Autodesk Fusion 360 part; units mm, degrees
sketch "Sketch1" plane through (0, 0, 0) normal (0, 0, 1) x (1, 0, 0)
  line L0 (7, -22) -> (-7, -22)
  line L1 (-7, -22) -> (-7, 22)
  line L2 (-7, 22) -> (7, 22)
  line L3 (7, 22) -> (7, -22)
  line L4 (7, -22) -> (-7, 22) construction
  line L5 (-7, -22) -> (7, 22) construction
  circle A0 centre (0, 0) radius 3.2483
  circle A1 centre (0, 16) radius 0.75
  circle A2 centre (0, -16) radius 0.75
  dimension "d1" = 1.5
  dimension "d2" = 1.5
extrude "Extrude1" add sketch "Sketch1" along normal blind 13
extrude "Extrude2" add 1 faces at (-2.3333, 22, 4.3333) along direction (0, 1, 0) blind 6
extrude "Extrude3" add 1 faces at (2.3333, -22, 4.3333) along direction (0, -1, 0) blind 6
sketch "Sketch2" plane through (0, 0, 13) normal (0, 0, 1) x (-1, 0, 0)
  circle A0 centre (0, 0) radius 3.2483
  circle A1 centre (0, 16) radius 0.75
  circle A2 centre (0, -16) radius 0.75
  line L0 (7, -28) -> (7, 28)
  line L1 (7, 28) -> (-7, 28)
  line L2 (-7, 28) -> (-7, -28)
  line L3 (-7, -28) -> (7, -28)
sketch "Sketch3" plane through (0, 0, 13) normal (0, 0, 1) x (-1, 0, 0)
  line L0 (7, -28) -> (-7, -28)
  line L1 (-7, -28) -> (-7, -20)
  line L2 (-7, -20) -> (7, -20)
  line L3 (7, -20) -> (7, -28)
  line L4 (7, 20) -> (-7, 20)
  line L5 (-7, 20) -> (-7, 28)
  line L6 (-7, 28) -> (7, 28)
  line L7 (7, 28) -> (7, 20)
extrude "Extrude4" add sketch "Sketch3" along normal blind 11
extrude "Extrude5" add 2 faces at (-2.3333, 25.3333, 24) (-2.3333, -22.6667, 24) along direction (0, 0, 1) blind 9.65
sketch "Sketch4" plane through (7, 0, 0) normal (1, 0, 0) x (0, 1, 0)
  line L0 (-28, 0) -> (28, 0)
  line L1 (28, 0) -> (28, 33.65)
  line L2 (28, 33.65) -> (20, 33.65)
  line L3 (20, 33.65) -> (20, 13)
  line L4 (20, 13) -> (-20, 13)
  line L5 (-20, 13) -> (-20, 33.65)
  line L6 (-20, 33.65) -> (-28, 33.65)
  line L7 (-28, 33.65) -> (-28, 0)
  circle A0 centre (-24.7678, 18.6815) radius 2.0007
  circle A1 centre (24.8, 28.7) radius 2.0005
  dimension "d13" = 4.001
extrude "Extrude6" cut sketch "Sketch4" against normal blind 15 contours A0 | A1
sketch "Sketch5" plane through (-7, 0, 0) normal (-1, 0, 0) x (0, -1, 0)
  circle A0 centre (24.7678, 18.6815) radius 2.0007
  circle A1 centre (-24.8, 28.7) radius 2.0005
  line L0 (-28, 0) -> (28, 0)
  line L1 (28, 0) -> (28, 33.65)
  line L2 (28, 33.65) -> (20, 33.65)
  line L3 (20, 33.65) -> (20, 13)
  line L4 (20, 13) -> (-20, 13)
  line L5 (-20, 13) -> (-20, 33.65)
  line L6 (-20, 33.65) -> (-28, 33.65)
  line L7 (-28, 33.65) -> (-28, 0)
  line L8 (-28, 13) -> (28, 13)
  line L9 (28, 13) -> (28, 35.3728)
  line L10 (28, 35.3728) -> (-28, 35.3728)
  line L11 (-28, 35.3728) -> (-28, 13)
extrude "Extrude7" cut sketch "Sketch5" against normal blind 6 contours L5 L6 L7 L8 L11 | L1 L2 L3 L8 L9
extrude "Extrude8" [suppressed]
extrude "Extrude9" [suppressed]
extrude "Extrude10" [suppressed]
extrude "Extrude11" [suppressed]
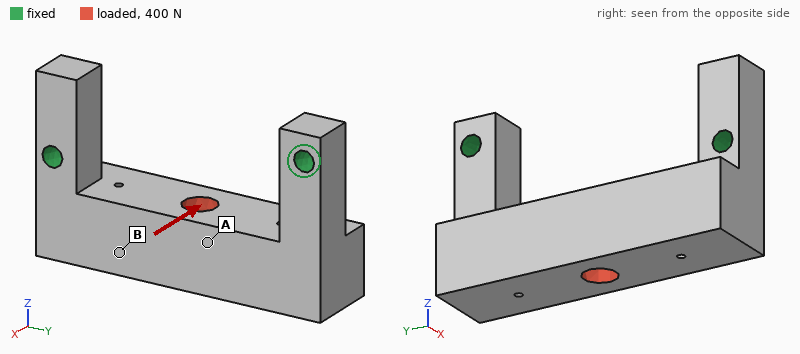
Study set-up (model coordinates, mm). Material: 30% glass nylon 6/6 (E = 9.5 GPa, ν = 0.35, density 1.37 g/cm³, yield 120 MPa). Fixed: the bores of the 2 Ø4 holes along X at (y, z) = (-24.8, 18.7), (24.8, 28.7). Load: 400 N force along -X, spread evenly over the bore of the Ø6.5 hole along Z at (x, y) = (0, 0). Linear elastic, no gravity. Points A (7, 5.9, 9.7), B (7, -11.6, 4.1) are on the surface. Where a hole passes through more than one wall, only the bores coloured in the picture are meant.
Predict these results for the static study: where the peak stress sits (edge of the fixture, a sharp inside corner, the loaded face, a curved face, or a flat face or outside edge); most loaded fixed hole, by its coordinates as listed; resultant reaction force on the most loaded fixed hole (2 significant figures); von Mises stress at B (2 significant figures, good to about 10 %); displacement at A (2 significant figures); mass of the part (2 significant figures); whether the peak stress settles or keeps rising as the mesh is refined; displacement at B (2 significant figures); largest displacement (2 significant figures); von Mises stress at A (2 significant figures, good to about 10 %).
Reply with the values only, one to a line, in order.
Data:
edge of the fixture
(-24.8, 18.7)
220 N
4.7 MPa
0.12 mm
17 g
keeps rising
0.11 mm
0.21 mm
7.8 MPa
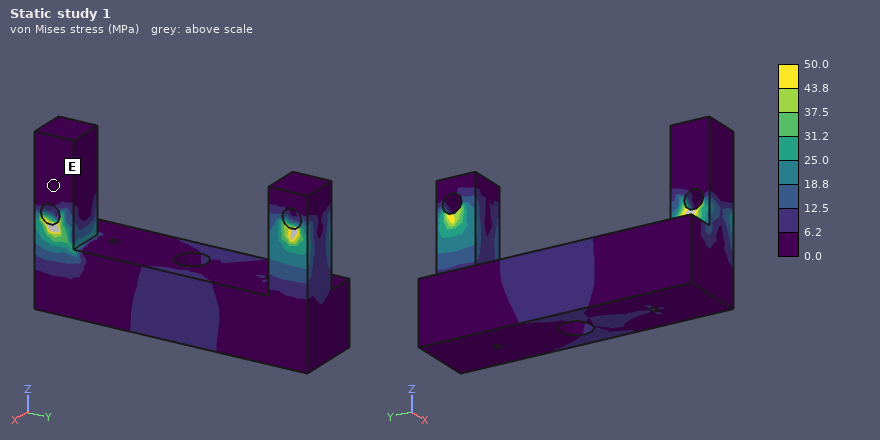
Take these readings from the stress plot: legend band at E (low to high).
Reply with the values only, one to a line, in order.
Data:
0.0 to 6.2 MPa
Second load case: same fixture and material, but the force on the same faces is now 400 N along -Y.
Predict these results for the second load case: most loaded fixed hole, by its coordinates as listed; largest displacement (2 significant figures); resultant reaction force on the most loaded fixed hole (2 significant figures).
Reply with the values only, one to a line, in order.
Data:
(-24.8, 18.7)
31 µm
310 N
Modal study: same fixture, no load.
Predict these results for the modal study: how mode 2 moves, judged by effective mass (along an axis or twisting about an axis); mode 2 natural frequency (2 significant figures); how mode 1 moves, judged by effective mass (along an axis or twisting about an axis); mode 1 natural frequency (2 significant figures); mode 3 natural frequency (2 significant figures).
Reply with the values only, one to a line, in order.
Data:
along Y
5200 Hz
along X
2400 Hz
6100 Hz
